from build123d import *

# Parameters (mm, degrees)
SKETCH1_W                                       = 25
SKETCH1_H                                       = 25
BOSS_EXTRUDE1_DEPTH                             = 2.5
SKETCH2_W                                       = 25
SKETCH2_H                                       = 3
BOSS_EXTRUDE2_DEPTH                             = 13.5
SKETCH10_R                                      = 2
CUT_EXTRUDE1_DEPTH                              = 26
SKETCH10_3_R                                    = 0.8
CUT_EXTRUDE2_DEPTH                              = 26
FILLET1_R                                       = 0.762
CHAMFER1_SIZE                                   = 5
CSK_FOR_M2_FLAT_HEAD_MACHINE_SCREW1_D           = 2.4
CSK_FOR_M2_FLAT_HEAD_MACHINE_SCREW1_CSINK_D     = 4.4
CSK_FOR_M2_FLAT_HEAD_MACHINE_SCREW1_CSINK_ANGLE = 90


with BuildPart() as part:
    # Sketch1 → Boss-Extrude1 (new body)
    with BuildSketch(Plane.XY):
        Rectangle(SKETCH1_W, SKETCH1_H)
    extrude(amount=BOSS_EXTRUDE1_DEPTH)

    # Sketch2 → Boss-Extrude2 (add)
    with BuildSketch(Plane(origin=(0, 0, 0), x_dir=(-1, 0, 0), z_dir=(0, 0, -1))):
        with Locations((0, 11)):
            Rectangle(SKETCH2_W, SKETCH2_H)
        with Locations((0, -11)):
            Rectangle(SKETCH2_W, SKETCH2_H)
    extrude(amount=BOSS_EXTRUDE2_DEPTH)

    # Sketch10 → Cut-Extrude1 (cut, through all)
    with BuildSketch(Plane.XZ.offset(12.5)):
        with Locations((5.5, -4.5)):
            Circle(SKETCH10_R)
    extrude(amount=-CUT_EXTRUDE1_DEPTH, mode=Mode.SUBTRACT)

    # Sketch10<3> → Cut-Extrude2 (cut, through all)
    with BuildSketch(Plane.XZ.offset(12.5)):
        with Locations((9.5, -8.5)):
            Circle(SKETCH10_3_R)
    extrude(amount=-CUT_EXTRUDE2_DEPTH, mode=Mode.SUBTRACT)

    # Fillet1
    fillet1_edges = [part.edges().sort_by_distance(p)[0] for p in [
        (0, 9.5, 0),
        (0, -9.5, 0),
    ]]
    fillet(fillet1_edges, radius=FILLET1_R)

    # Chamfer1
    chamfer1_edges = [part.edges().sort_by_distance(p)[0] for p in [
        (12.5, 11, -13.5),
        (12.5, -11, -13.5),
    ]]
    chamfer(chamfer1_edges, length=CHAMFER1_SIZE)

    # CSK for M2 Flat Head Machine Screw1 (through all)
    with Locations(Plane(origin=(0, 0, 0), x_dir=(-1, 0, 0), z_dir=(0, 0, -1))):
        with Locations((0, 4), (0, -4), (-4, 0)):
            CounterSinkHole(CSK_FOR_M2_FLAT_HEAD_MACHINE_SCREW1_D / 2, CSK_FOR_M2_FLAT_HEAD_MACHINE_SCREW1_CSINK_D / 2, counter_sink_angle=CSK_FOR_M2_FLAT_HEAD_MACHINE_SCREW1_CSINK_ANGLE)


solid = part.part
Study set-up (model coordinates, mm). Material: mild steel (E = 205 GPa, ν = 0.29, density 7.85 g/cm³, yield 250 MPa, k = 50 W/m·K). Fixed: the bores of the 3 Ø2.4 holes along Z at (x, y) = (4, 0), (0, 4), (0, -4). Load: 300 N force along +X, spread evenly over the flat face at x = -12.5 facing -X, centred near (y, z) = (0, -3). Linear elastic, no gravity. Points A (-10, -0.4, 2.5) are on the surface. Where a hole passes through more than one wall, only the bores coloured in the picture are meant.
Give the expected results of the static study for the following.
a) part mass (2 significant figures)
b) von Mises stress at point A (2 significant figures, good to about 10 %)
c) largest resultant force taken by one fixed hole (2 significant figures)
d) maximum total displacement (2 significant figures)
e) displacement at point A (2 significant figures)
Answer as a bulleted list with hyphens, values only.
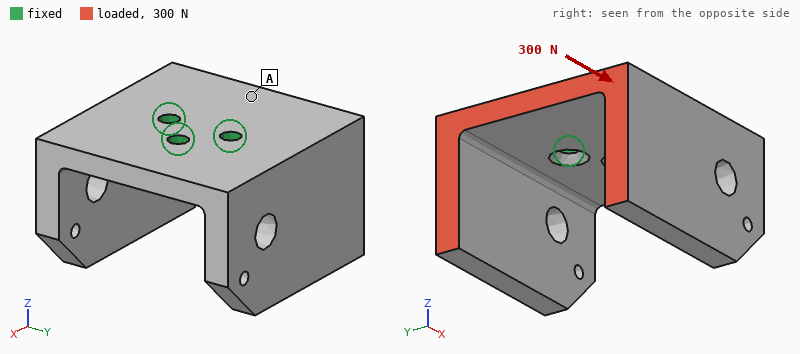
- 27 g
- 9.5 MPa
- 150 N
- 11 µm
- 4.3 µm
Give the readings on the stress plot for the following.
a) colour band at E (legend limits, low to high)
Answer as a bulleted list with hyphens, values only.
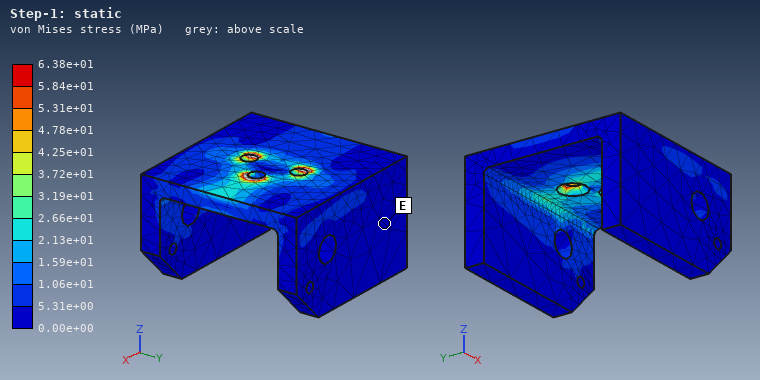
- 0.00e+00 to 5.31e+00 MPa
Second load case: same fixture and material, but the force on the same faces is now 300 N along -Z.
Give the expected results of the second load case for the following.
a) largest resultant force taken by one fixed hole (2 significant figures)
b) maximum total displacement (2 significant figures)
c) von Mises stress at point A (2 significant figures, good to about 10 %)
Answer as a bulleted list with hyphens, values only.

- 370 N
- 31 µm
- 19 MPa
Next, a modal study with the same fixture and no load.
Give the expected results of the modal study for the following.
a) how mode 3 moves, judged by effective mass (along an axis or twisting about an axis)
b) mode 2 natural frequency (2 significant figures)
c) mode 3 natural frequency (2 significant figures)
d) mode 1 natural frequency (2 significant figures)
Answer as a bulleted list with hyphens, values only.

- along X
- 4900 Hz
- 5400 Hz
- 4700 Hz
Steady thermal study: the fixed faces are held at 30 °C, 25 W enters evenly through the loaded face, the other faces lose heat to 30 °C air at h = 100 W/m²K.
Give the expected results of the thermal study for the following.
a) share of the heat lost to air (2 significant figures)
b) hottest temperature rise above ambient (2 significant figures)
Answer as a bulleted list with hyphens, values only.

- 33 %
- 66 K
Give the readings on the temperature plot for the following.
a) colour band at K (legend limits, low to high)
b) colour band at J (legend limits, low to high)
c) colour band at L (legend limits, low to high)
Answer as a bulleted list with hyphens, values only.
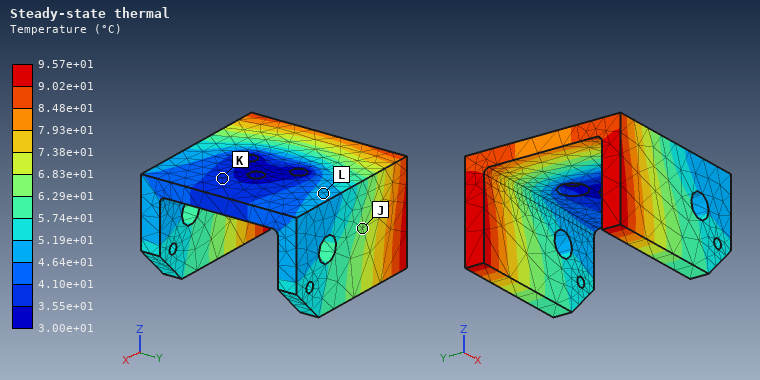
- 3.55e+01 to 4.10e+01 °C
- 6.29e+01 to 6.83e+01 °C
- 4.64e+01 to 5.19e+01 °C
